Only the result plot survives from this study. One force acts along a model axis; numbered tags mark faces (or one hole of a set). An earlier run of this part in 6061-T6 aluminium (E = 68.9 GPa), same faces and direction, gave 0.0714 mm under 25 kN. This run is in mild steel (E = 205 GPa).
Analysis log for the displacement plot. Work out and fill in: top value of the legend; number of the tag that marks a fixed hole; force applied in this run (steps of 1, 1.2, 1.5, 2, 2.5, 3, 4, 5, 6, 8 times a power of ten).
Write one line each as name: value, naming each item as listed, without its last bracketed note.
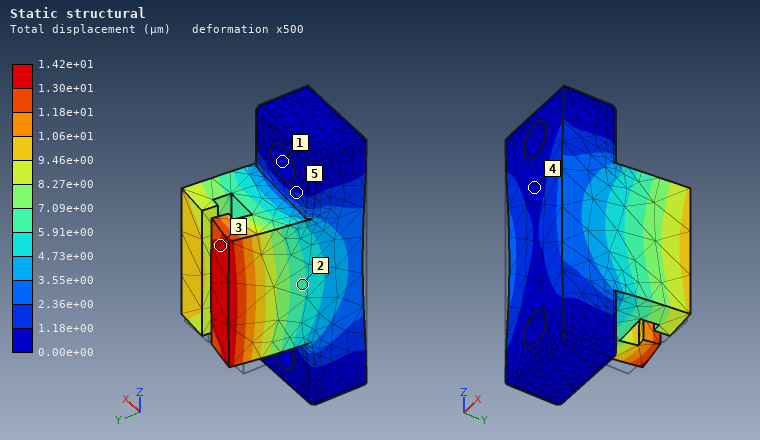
top value of the legend: 1.42e+01 µm
number of the tag that marks a fixed hole: 1
force applied in this run: 15 kN
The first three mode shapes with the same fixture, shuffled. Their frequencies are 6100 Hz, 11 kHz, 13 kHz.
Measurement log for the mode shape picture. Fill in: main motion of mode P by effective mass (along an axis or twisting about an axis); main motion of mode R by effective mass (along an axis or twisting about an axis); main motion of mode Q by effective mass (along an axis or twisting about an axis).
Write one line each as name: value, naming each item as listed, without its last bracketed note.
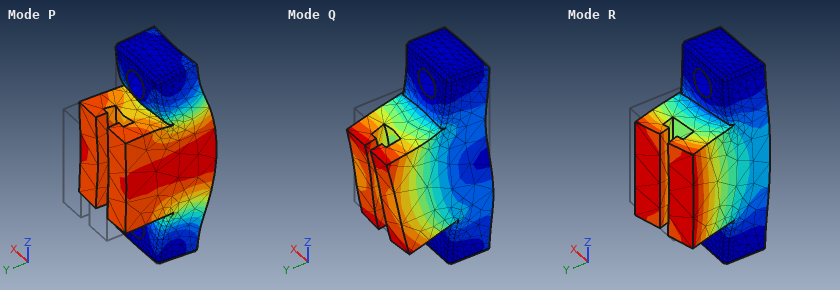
main motion of mode P by effective mass: along Y
main motion of mode R by effective mass: along X
main motion of mode Q by effective mass: along Z
